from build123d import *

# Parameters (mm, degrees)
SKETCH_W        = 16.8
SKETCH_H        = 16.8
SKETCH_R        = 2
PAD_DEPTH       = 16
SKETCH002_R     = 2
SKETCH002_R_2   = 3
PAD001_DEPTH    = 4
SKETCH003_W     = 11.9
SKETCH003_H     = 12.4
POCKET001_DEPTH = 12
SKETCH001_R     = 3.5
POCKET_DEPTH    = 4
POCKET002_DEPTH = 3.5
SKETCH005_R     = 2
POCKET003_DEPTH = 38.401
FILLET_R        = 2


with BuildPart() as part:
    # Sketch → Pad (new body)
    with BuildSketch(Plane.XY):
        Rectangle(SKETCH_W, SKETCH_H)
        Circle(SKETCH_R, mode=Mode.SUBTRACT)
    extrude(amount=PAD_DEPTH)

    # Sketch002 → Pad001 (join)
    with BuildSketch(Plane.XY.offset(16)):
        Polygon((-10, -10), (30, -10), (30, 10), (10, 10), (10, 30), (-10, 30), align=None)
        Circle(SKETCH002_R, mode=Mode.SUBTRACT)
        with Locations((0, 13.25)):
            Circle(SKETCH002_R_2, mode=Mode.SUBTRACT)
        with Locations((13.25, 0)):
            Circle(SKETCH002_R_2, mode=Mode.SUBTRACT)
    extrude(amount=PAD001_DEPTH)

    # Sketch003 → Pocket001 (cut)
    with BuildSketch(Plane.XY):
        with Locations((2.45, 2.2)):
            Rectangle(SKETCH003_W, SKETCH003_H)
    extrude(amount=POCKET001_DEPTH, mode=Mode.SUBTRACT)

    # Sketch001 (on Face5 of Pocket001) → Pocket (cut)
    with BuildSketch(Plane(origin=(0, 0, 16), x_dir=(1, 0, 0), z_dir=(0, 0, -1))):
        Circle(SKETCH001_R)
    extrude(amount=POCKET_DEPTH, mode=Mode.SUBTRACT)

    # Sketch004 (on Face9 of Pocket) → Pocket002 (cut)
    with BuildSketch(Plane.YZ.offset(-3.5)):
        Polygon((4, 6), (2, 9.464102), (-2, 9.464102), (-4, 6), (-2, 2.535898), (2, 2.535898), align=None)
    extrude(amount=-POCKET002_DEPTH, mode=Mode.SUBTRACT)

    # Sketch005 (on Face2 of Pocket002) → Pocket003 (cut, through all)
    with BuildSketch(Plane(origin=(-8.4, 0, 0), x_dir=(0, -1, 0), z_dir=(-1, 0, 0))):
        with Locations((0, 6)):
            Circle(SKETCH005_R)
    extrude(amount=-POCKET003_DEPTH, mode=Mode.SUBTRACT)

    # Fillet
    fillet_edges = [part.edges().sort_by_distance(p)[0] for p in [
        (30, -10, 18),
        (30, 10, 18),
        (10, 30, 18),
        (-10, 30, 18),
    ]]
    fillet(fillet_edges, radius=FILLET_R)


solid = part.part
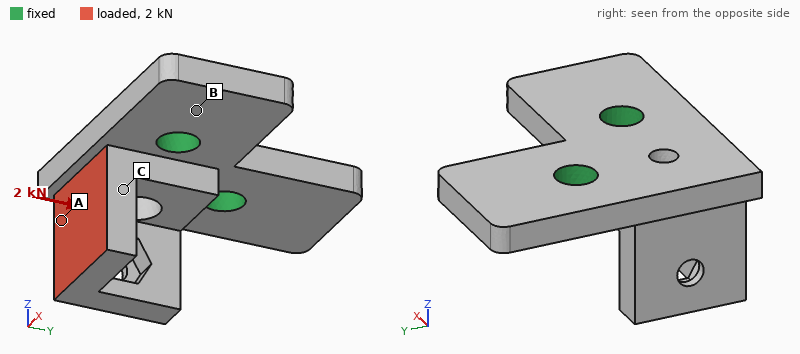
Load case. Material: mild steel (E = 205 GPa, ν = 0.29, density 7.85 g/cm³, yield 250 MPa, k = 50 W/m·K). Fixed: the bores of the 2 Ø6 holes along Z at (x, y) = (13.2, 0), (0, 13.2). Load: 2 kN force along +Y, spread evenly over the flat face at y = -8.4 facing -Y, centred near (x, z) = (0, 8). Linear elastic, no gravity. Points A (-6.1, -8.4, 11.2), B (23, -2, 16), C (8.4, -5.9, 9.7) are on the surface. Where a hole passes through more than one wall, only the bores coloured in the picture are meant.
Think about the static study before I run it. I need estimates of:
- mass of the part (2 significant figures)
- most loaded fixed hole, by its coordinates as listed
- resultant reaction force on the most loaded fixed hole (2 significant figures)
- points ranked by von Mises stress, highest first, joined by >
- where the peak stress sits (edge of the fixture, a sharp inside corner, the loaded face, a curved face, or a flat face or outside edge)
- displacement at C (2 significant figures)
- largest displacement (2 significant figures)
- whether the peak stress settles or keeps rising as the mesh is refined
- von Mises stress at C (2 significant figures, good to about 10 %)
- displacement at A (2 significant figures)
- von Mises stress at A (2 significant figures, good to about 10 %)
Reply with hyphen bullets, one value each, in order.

- 54 g
- (0, 13.2)
- 1.7 kN
- C > A > B
- edge of the fixture
- 20 µm
- 53 µm
- keeps rising
- 68 MPa
- 34 µm
- 43 MPa
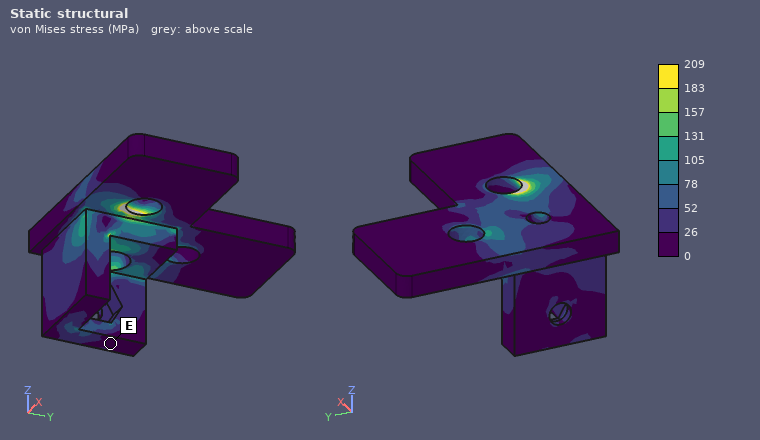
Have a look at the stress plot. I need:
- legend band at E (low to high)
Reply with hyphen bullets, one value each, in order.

- 0 to 26 MPa
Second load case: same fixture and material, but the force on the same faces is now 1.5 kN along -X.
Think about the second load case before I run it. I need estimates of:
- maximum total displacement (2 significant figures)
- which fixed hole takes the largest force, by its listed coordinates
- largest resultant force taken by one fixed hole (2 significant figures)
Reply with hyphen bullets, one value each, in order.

- 42 µm
- (13.2, 0)
- 1.8 kN
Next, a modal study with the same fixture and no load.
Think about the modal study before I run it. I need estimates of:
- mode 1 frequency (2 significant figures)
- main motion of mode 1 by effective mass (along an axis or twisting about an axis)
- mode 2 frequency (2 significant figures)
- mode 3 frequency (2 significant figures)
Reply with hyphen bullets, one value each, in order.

- 6600 Hz
- along Z
- 13 kHz
- 13 kHz
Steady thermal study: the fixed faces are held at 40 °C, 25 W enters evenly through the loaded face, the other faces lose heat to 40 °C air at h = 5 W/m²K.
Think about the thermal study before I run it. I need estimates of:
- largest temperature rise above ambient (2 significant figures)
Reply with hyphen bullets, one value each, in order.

- 82 K
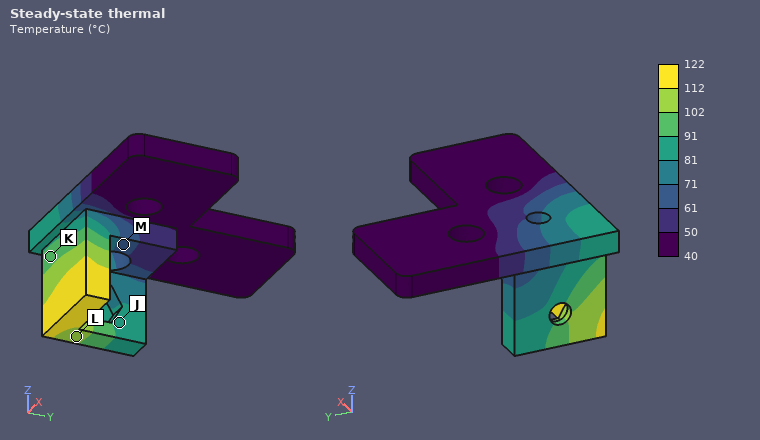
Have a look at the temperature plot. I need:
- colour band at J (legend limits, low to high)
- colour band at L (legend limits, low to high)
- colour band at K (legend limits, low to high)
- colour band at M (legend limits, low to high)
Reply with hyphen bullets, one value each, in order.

- 81 to 91 °C
- 102 to 112 °C
- 91 to 102 °C
- 61 to 71 °C
